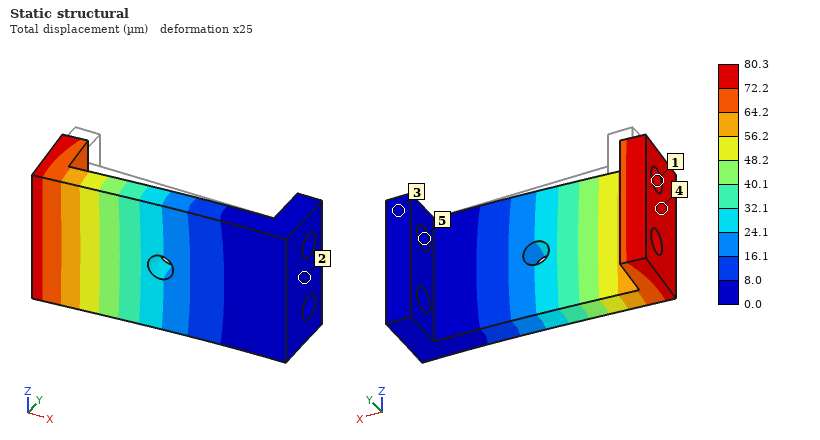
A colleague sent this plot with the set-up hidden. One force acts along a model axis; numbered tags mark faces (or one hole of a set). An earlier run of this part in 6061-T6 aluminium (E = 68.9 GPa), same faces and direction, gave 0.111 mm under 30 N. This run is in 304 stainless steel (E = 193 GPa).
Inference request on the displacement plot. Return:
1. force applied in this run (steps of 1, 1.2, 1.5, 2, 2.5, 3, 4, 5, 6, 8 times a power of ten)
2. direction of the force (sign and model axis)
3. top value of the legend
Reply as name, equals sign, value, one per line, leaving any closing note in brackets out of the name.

force applied in this run = 60 N
direction of the force = -Y
top value of the legend = 80.3 µm
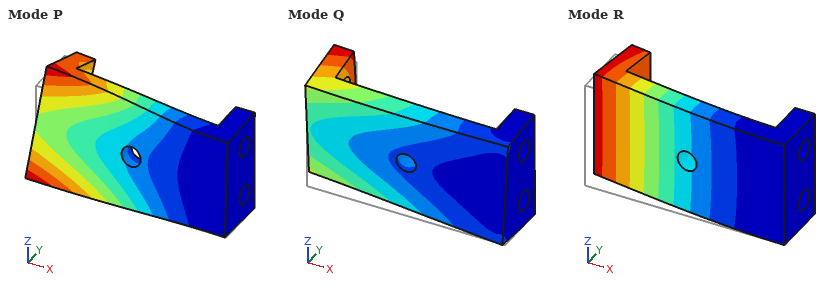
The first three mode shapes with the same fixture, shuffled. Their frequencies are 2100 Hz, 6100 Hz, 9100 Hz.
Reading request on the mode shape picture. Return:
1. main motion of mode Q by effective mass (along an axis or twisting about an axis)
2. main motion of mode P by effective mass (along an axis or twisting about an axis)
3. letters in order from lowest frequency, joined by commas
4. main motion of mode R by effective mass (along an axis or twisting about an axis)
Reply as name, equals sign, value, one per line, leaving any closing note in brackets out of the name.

main motion of mode Q by effective mass = along Z
main motion of mode P by effective mass = along Z
letters in order from lowest frequency, joined by commas = R, Q, P
main motion of mode R by effective mass = along Y
